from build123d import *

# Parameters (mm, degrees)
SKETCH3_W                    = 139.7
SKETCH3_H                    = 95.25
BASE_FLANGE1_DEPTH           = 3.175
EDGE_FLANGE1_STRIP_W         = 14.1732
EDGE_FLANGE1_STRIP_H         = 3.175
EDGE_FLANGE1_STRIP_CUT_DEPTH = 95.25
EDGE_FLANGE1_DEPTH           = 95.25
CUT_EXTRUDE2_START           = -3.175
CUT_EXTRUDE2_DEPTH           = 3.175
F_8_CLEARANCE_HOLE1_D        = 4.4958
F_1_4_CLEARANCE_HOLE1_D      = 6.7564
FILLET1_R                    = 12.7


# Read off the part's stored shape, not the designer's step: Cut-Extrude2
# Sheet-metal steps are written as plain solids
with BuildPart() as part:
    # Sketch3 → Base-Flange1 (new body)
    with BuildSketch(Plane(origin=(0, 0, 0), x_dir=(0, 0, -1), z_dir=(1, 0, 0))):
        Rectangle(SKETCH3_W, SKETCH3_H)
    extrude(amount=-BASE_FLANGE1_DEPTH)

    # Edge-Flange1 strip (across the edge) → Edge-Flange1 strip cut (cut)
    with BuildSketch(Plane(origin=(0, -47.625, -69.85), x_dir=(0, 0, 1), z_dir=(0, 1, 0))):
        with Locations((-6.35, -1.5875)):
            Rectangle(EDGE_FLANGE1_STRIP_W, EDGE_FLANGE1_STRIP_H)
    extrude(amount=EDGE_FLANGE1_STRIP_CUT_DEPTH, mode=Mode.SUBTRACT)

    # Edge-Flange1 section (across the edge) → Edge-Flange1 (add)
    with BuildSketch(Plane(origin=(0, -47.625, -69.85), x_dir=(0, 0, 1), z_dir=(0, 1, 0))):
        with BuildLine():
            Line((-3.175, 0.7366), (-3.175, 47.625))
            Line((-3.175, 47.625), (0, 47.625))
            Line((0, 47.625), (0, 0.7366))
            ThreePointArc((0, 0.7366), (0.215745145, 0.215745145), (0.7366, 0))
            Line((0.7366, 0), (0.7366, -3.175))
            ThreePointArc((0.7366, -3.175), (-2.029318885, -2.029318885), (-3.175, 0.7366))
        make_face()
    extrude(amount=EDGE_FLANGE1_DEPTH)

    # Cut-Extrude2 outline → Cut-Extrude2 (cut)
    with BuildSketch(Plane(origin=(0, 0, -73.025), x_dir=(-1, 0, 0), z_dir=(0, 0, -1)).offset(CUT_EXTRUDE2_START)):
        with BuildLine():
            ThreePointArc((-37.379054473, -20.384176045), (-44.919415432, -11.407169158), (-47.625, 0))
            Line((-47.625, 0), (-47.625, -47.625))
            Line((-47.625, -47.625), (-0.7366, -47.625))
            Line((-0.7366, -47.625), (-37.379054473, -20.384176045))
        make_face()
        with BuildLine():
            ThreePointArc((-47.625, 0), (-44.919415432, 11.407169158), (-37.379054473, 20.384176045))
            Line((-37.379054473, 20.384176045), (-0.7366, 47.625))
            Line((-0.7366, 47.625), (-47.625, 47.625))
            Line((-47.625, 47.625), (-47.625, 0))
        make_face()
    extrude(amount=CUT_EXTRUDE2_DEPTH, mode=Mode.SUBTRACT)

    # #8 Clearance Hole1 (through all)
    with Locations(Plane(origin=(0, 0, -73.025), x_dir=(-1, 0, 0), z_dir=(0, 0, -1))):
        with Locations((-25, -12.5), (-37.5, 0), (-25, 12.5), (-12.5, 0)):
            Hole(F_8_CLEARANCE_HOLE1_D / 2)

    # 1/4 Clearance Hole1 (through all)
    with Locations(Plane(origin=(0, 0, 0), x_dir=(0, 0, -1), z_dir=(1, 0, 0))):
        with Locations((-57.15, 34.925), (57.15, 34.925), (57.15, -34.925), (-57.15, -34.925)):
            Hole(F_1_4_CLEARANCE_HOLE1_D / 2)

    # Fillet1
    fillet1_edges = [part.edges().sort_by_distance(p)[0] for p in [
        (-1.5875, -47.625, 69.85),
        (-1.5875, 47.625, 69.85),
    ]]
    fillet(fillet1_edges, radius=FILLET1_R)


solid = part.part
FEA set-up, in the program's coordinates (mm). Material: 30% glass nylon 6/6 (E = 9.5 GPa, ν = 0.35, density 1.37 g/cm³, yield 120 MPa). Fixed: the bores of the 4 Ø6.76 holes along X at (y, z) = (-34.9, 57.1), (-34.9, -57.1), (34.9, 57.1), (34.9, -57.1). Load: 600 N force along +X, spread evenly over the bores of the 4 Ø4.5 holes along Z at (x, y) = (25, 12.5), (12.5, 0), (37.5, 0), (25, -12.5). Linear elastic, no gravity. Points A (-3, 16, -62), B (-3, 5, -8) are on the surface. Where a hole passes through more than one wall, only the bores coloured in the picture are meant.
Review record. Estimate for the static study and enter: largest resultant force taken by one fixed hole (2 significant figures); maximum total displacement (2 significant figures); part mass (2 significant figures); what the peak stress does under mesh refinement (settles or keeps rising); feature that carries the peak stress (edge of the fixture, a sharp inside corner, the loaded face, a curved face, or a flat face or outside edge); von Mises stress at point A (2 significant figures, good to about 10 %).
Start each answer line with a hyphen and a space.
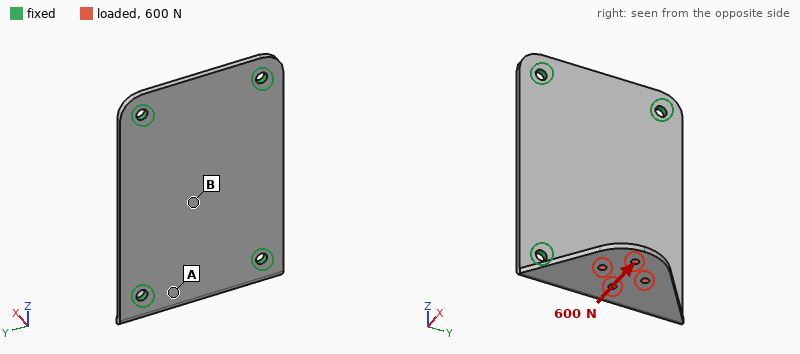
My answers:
- 330 N
- 1.2 mm
- 70 g
- keeps rising
- edge of the fixture
- 14 MPa
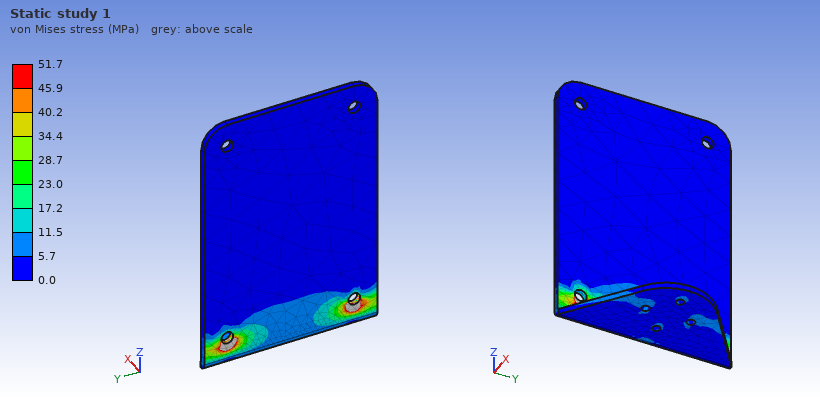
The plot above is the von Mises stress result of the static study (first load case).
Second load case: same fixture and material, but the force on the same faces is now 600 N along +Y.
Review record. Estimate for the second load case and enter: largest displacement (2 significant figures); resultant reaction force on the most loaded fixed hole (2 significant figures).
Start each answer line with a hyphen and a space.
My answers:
- 0.33 mm
- 390 N
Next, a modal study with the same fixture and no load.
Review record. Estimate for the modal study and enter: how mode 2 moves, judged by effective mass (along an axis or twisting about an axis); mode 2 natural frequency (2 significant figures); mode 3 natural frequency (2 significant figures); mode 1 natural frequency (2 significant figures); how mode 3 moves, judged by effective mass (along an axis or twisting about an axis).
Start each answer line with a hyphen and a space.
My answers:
- along X
- 640 Hz
- 880 Hz
- 560 Hz
- twisting about Z
